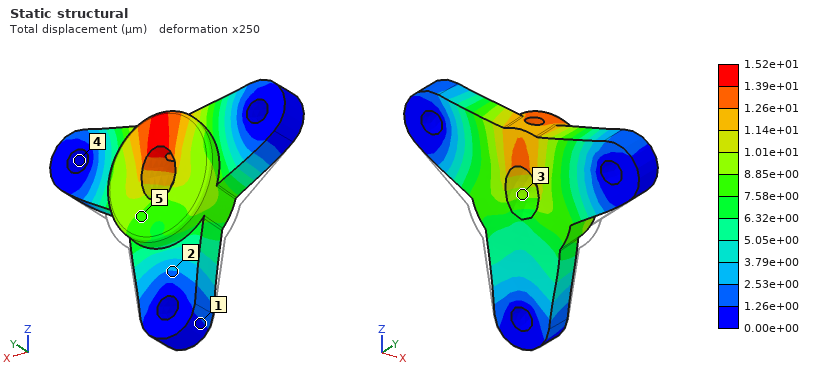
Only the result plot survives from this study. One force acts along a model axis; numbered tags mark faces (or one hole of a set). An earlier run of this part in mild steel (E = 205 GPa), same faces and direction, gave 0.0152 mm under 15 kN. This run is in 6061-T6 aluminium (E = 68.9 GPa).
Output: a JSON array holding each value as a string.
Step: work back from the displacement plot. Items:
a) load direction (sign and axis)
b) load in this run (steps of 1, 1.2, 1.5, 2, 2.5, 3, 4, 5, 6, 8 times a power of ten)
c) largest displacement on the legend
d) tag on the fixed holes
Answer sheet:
["+Z", "5 kN", "1.52e+01 µm", "4"]
